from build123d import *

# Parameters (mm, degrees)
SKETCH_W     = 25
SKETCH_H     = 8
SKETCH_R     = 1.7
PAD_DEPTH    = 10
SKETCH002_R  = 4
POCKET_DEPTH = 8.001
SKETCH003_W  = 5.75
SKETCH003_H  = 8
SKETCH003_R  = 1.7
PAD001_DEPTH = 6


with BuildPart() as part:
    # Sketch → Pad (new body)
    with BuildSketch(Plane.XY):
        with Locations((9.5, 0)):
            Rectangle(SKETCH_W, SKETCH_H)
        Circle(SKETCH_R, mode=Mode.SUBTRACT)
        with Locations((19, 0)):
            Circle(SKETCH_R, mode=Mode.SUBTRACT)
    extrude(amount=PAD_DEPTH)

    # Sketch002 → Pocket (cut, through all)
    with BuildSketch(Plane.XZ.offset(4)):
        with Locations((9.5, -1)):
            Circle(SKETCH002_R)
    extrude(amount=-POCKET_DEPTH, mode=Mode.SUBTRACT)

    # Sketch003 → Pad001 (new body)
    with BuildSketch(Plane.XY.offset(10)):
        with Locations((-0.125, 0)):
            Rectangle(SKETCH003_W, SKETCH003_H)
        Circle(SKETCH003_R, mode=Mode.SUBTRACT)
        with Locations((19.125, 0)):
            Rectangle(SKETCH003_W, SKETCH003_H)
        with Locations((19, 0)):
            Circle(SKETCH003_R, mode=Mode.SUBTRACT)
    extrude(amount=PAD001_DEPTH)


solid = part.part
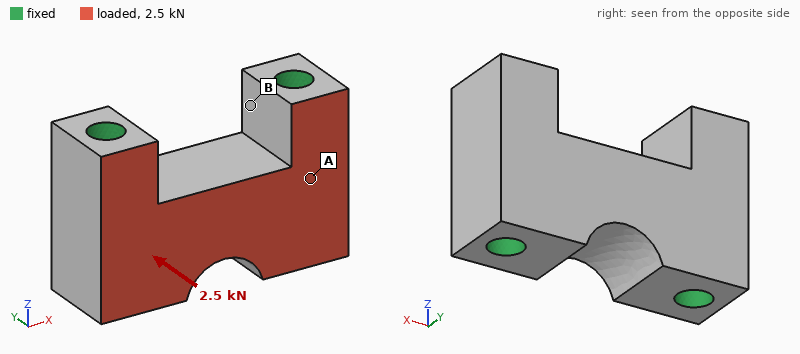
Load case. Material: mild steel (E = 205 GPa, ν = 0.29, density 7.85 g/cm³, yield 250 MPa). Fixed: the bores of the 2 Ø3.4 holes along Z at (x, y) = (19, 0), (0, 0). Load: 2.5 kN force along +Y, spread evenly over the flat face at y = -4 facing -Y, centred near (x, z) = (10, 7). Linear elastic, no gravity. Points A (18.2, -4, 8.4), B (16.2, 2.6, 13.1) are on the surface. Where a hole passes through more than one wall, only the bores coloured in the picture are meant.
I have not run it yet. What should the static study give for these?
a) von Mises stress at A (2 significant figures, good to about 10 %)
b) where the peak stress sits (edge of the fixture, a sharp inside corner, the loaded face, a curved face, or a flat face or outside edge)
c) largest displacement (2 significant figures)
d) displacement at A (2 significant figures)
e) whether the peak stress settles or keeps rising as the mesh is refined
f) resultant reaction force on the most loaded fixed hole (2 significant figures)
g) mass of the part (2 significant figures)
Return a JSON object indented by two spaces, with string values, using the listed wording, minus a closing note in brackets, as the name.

{
  "von Mises stress at A": "16 MPa",
  "where the peak stress sits": "edge of the fixture",
  "largest displacement": "1.0 µm",
  "displacement at A": "0.22 µm",
  "whether the peak stress settles or keeps rising as the mesh is refined": "keeps rising",
  "resultant reaction force on the most loaded fixed hole": "1.3 kN",
  "mass of the part": "17 g"
}
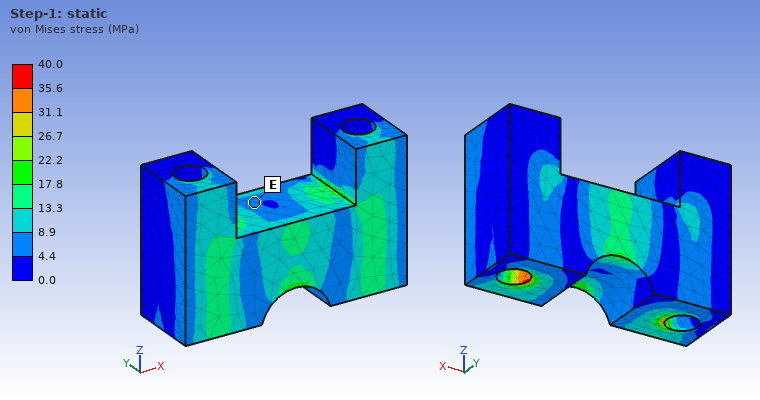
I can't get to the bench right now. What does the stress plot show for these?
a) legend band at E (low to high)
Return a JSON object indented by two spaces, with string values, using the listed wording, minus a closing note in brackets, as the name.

{
  "legend band at E": "4.4 to 8.9 MPa"
}
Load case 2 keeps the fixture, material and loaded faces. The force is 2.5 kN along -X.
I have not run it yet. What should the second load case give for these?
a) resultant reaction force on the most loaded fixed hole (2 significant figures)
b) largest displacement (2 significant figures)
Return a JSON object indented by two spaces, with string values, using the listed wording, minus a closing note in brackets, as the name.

{
  "resultant reaction force on the most loaded fixed hole": "1.3 kN",
  "largest displacement": "0.73 µm"
}
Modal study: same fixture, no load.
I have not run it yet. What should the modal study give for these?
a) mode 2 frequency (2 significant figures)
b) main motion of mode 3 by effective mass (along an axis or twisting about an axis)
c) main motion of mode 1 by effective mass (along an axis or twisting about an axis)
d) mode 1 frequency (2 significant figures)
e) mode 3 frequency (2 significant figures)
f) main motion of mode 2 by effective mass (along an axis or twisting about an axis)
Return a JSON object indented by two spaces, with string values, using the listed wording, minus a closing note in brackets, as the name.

{
  "mode 2 frequency": "84 kHz",
  "main motion of mode 3 by effective mass": "twisting about X",
  "main motion of mode 1 by effective mass": "along Y",
  "mode 1 frequency": "70 kHz",
  "mode 3 frequency": "100 kHz",
  "main motion of mode 2 by effective mass": "along Z"
}
